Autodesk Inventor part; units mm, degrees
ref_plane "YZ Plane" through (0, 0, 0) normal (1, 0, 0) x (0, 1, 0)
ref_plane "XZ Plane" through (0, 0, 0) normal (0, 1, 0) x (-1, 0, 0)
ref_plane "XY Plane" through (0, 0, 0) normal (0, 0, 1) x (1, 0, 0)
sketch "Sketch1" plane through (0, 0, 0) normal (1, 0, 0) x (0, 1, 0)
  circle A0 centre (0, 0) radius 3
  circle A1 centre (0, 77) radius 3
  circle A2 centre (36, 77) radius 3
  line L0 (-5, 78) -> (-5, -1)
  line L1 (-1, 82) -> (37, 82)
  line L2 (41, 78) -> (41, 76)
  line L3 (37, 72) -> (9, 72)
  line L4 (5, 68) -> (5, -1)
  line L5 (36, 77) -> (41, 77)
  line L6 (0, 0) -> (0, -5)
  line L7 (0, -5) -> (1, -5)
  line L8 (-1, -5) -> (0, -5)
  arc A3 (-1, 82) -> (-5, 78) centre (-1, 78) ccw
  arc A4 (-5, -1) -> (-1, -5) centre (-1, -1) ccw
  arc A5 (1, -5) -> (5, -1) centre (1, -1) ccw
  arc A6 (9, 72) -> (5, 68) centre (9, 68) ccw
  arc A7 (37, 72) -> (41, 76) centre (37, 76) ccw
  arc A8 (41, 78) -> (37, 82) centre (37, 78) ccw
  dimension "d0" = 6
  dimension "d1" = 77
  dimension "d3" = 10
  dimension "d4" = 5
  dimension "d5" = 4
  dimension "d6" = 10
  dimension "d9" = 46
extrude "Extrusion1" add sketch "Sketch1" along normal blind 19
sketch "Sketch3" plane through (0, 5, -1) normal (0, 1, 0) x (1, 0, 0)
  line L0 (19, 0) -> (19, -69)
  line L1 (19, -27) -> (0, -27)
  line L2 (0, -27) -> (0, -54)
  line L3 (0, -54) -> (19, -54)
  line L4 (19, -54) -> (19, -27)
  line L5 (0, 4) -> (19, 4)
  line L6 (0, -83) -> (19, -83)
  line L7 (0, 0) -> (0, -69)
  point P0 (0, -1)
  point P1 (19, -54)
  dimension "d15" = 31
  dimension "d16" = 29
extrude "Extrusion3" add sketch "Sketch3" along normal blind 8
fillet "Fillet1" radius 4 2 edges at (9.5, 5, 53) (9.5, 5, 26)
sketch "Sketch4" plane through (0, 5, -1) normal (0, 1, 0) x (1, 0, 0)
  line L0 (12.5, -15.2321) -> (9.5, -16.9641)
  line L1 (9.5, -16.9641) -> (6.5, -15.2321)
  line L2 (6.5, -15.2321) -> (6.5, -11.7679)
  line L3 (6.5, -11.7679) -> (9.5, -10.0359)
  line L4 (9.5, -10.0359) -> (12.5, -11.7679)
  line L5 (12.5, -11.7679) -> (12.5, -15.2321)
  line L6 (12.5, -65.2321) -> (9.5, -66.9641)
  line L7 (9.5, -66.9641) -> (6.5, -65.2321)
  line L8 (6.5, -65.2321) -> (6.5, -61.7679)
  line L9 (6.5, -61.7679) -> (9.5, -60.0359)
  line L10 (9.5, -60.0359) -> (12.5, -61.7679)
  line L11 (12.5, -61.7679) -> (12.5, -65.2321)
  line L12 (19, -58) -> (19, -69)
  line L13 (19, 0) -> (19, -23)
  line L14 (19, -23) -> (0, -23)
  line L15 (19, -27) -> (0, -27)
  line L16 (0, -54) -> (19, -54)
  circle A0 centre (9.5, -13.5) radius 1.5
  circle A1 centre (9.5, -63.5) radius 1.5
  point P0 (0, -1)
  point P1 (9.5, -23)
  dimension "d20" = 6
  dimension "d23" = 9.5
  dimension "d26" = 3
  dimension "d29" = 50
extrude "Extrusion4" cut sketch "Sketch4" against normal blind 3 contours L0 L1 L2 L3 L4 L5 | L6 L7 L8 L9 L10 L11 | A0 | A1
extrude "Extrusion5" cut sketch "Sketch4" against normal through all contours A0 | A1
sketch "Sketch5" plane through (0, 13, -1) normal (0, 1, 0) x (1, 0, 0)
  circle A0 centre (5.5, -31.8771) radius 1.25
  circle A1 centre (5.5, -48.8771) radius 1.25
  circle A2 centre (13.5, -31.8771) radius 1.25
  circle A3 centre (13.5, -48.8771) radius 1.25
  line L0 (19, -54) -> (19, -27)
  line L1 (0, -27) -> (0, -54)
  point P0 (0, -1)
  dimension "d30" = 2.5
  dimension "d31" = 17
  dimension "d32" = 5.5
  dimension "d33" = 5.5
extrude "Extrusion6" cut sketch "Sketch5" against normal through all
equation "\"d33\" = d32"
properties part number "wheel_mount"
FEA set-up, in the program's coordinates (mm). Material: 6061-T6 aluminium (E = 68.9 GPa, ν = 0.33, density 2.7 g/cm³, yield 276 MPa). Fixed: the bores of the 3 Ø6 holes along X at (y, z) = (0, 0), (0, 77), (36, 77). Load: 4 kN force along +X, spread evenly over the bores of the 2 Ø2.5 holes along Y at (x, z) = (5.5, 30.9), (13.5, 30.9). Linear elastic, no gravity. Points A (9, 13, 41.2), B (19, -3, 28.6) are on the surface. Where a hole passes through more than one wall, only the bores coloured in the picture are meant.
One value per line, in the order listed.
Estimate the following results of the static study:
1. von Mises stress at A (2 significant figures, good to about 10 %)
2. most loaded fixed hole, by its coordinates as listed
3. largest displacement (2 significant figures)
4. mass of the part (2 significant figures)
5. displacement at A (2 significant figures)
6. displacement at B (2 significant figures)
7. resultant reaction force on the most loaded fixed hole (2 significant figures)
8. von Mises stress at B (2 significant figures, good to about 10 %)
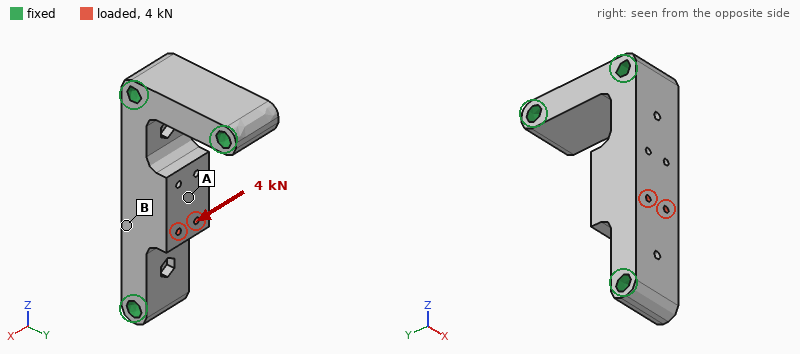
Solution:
14 MPa
(0, 0)
62 µm
68 g
54 µm
30 µm
2.5 kN
51 MPa
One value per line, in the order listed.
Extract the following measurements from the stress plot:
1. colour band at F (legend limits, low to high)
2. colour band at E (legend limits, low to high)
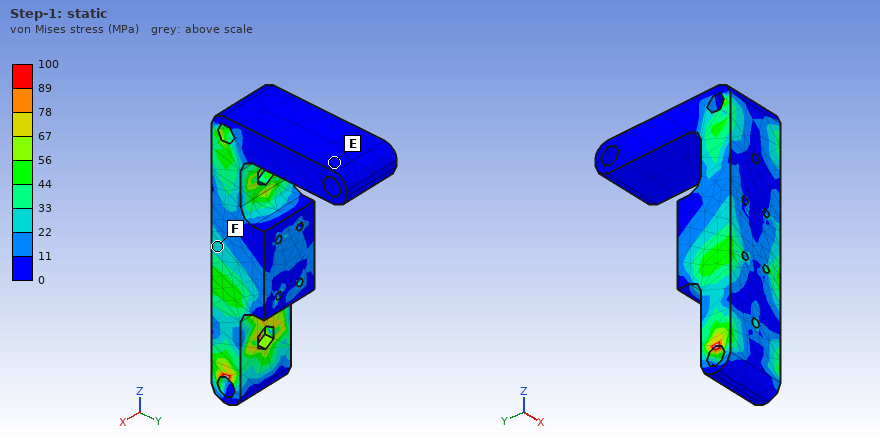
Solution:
22 to 33 MPa
0 to 11 MPa
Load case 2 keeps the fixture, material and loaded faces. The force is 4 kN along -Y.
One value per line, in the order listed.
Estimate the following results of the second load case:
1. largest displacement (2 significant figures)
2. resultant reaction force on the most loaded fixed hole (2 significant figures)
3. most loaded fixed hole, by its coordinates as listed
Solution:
55 µm
2.7 kN
(0, 0)
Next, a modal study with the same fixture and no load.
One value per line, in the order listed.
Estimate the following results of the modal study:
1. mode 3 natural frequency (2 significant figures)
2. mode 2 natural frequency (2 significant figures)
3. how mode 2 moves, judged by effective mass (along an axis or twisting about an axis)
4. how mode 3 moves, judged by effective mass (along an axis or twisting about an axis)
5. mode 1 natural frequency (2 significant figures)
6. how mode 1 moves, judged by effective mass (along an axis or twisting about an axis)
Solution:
14 kHz
9000 Hz
along X
along X
8500 Hz
along Y
